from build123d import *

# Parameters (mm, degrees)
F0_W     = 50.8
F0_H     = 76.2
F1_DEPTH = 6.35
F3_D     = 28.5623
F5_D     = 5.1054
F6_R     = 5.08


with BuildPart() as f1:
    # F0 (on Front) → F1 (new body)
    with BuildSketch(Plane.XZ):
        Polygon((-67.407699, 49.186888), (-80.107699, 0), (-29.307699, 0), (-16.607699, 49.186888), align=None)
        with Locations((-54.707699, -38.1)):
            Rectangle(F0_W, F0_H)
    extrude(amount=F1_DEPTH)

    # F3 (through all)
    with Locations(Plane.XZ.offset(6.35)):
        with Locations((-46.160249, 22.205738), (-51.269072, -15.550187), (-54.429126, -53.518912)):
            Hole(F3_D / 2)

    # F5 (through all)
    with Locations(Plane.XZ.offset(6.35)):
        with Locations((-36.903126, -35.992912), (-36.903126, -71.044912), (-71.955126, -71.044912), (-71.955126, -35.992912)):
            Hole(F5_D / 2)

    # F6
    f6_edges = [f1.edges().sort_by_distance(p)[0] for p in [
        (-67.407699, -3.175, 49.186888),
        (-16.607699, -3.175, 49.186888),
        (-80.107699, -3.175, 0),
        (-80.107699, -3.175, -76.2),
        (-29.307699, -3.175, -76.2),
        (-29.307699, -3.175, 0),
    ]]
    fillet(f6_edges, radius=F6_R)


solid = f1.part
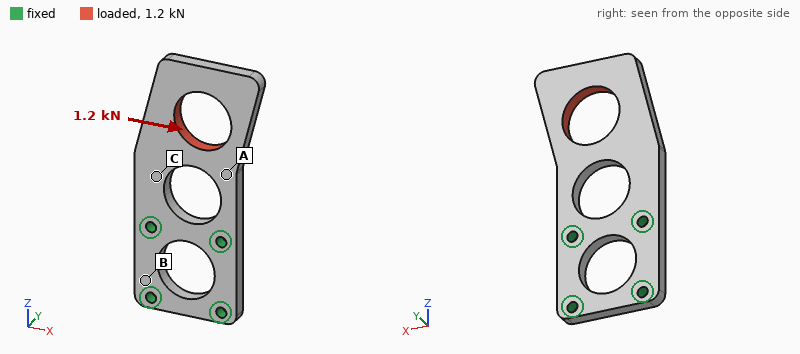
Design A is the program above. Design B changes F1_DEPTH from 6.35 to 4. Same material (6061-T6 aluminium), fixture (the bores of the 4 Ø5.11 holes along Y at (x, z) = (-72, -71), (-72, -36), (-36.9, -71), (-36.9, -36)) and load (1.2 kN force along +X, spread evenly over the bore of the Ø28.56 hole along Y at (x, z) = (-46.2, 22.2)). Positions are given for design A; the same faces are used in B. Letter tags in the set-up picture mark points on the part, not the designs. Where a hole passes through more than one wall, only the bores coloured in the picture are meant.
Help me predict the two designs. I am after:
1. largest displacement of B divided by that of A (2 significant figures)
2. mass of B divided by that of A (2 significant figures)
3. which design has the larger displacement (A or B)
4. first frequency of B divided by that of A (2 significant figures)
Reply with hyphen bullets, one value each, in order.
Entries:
- 1.6
- 0.63
- B
- 0.64
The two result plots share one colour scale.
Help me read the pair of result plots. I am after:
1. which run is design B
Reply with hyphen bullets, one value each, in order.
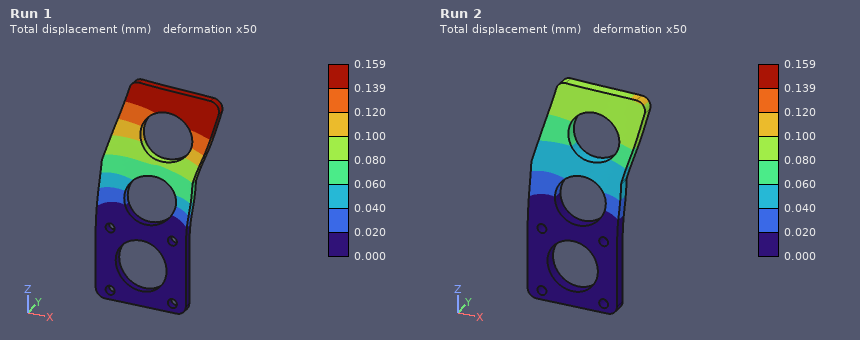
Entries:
- Run 1
